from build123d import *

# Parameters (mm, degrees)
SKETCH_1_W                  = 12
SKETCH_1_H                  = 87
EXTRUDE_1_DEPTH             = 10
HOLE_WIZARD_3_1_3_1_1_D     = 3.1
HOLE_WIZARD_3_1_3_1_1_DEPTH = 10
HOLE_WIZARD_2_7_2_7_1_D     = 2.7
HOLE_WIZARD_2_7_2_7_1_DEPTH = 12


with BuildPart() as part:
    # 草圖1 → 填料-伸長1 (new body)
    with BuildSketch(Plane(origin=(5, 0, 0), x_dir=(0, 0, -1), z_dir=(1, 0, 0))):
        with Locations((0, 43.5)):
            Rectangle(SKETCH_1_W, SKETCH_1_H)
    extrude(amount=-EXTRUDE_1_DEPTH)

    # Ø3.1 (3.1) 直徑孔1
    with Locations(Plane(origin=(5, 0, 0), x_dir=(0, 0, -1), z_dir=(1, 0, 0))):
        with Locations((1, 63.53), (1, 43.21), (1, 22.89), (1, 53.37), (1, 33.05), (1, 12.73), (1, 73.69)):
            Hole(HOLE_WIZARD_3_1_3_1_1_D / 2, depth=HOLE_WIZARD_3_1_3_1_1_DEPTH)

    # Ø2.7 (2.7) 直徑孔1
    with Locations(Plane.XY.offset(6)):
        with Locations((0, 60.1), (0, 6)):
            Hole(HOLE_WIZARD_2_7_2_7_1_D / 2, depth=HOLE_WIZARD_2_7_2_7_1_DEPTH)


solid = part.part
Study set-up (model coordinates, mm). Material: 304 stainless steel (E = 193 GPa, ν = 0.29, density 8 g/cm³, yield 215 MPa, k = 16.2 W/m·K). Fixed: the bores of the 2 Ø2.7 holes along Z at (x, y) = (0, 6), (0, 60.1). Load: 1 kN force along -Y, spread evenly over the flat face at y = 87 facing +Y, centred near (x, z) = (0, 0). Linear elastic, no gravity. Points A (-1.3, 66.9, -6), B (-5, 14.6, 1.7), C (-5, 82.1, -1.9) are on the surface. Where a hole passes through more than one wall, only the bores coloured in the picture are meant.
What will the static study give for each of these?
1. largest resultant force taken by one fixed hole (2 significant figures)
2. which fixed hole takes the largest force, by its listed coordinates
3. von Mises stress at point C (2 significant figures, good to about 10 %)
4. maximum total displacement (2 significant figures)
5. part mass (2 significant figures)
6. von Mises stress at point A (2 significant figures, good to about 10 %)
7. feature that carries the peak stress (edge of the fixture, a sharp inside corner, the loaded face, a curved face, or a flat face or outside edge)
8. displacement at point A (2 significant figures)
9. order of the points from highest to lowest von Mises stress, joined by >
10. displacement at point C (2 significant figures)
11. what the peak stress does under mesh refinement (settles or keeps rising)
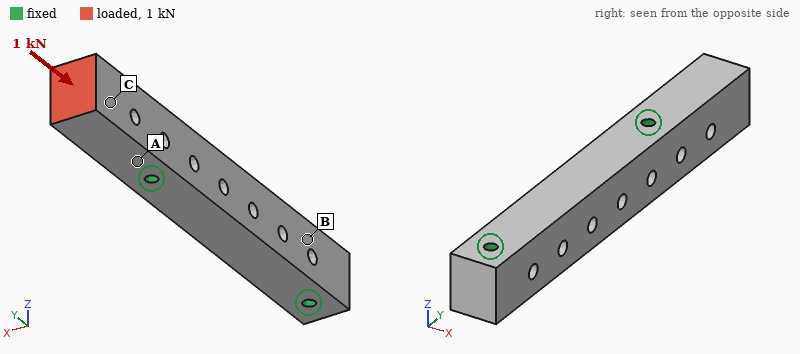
970 N
(0, 60.1)
7.9 MPa
1.5 µm
78 g
12 MPa
edge of the fixture
0.44 µm
A > C > B
1.2 µm
keeps rising
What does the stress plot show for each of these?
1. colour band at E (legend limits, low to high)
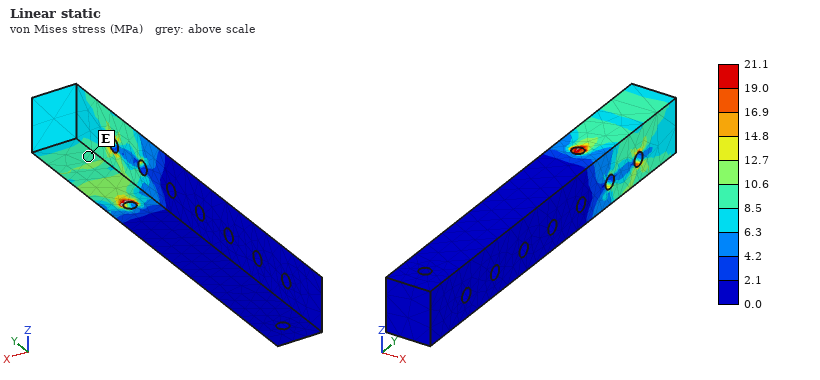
8.5 to 10.6 MPa
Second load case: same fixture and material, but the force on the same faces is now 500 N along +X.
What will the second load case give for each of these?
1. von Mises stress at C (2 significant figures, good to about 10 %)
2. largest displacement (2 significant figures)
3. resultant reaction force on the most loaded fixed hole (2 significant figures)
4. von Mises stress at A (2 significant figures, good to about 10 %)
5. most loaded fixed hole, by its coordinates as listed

12 MPa
33 µm
600 N
22 MPa
(0, 60.1)
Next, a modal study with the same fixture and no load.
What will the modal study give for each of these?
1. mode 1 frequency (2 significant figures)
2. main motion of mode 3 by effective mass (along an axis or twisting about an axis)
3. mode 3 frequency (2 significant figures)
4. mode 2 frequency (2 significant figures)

7100 Hz
along X
12 kHz
11 kHz
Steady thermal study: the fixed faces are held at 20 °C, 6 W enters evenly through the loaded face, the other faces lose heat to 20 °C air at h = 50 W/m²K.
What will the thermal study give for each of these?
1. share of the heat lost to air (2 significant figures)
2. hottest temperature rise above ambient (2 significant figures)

36 %
70 K
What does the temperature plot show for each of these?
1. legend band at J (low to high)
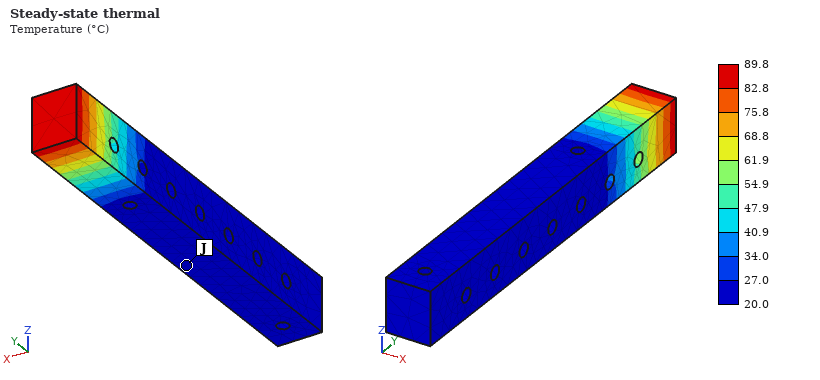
20.0 to 27.0 °C
